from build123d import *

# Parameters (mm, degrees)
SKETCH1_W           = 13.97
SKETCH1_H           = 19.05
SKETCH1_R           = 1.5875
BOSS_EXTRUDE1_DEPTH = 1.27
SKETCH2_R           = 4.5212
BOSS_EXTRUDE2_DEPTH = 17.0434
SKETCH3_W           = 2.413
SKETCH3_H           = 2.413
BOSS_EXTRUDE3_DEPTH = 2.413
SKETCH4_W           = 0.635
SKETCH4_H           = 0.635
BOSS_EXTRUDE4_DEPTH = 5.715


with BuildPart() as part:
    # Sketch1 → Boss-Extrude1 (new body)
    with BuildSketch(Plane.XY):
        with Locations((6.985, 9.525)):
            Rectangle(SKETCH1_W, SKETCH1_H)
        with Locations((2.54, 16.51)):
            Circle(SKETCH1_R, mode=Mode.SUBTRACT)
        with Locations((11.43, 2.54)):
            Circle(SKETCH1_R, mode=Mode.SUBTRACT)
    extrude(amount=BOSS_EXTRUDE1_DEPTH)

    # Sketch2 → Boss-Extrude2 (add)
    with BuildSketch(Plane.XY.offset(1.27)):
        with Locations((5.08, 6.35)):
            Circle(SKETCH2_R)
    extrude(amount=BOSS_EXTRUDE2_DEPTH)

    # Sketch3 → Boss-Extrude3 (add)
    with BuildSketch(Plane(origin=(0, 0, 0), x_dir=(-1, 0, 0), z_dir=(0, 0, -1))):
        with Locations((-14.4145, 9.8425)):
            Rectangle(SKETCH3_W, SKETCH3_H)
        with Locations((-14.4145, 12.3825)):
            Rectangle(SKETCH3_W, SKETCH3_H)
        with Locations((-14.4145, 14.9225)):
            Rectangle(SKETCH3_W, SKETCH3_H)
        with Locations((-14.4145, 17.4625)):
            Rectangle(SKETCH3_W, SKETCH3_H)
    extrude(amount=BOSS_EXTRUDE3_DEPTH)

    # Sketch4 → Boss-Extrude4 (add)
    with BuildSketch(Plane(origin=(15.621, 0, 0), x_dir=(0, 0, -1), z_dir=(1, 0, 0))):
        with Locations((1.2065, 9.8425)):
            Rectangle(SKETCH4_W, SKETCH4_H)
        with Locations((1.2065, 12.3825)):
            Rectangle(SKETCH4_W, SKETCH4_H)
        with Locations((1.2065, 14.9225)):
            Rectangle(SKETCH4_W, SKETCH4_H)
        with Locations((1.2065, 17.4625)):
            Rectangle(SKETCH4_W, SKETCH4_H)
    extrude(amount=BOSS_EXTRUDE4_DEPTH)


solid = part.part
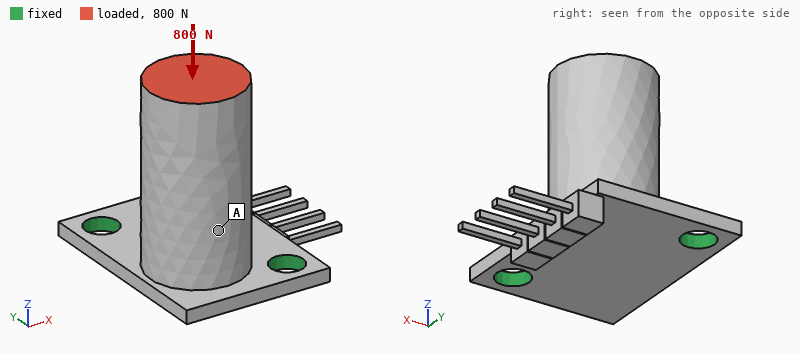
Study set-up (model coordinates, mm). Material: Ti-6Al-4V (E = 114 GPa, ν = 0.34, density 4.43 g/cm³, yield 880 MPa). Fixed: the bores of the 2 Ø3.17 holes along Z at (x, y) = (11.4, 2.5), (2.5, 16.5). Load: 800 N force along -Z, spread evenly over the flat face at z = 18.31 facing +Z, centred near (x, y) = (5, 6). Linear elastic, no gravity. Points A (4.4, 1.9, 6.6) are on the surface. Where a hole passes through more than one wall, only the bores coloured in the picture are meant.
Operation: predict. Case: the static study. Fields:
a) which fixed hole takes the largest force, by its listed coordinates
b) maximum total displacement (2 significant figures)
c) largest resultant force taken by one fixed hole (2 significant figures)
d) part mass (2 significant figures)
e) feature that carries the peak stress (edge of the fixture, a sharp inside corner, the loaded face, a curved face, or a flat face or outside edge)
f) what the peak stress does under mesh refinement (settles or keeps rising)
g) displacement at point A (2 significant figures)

(11.4, 2.5)
0.20 mm
500 N
6.5 g
edge of the fixture
keeps rising
0.088 mm
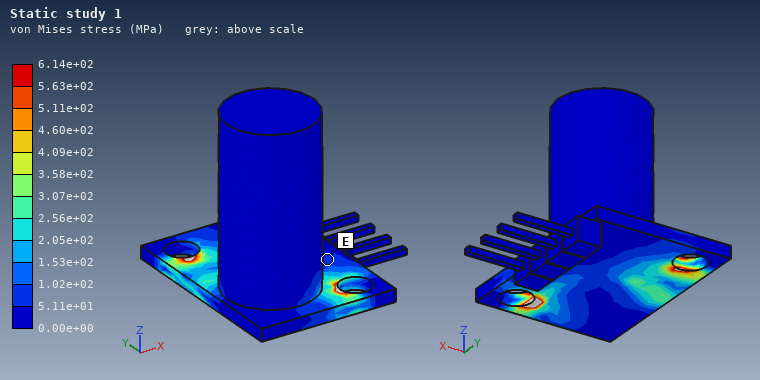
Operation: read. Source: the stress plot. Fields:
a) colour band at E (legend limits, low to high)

5.11e+01 to 1.02e+02 MPa
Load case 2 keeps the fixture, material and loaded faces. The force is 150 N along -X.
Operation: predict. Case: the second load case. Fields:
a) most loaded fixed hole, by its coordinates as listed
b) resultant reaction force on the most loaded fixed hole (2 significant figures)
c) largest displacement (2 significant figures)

(11.4, 2.5)
180 N
0.22 mm
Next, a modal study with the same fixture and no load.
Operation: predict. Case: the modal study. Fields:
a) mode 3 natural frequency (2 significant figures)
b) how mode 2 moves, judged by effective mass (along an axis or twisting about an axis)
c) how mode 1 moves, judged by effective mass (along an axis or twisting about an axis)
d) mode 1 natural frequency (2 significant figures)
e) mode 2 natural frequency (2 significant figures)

8000 Hz
along Y
along X
2900 Hz
6200 Hz
